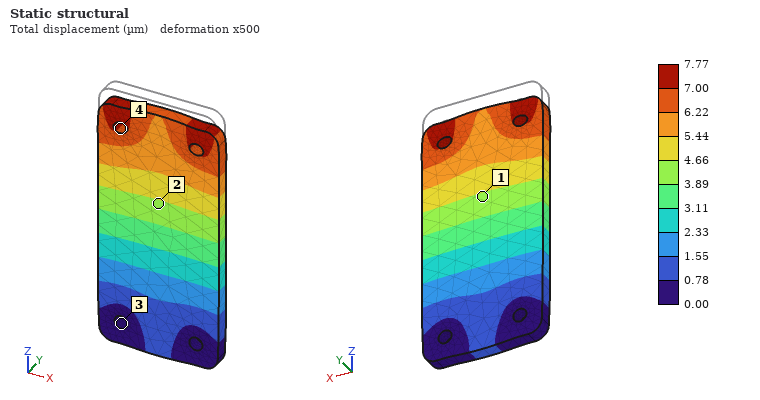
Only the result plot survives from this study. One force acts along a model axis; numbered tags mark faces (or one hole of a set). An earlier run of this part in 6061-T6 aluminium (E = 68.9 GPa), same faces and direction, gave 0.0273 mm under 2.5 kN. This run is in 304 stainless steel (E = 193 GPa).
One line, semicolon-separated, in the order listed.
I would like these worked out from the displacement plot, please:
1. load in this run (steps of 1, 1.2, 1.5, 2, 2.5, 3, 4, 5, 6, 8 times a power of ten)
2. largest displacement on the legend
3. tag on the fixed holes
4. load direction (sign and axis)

2 kN; 7.77 µm; 3; -Z
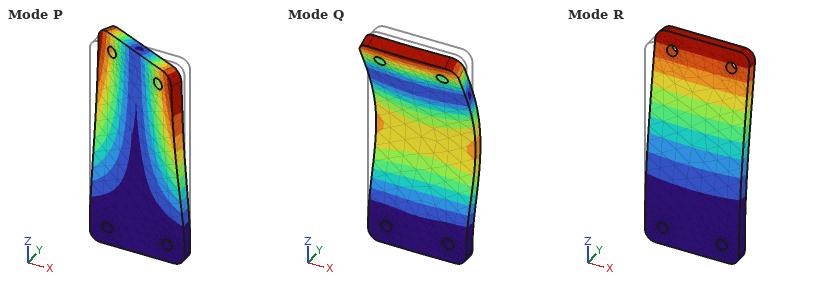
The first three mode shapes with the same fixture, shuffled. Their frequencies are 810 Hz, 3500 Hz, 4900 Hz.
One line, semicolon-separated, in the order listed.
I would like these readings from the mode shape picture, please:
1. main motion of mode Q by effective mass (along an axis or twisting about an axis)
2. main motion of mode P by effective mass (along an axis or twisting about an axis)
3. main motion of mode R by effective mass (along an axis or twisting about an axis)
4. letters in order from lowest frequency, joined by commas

along Y; twisting about Z; along Y; R, P, Q
